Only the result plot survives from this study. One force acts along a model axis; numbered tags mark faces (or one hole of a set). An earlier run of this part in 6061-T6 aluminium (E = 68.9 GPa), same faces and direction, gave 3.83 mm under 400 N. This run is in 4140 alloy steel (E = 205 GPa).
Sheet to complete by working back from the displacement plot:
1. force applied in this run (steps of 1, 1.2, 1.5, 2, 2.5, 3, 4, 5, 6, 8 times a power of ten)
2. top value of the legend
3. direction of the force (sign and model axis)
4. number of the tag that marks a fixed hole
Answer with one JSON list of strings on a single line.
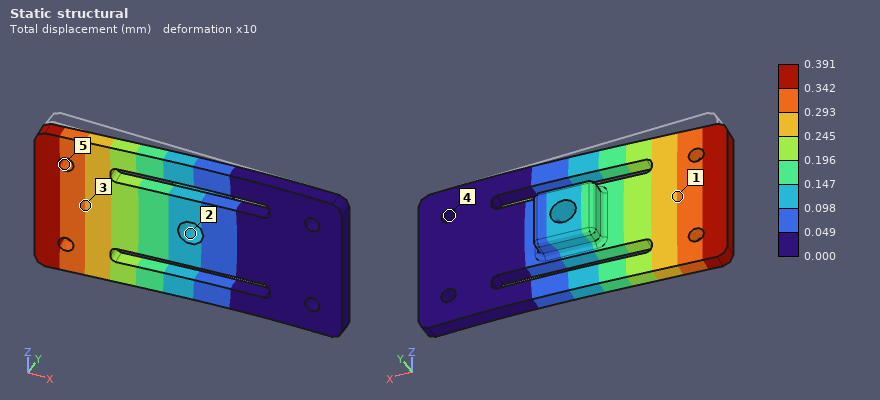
["120 N", "0.391 mm", "-Y", "4"]
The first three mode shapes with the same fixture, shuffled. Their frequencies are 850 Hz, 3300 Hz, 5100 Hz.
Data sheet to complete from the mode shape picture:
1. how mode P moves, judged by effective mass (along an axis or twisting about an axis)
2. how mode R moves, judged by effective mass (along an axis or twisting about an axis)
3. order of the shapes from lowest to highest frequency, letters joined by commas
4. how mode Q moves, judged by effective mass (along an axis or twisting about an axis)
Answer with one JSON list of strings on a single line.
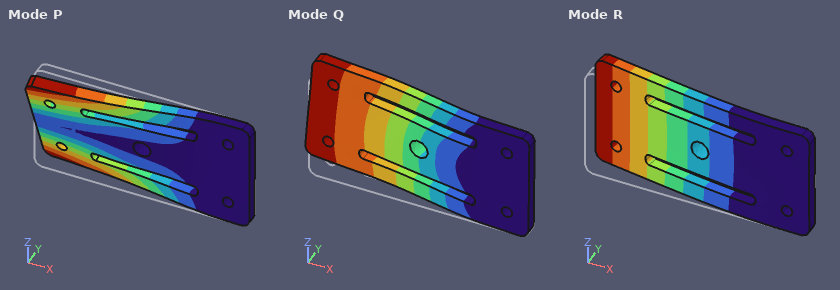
["twisting about X", "along Y", "R, P, Q", "along Z"]
